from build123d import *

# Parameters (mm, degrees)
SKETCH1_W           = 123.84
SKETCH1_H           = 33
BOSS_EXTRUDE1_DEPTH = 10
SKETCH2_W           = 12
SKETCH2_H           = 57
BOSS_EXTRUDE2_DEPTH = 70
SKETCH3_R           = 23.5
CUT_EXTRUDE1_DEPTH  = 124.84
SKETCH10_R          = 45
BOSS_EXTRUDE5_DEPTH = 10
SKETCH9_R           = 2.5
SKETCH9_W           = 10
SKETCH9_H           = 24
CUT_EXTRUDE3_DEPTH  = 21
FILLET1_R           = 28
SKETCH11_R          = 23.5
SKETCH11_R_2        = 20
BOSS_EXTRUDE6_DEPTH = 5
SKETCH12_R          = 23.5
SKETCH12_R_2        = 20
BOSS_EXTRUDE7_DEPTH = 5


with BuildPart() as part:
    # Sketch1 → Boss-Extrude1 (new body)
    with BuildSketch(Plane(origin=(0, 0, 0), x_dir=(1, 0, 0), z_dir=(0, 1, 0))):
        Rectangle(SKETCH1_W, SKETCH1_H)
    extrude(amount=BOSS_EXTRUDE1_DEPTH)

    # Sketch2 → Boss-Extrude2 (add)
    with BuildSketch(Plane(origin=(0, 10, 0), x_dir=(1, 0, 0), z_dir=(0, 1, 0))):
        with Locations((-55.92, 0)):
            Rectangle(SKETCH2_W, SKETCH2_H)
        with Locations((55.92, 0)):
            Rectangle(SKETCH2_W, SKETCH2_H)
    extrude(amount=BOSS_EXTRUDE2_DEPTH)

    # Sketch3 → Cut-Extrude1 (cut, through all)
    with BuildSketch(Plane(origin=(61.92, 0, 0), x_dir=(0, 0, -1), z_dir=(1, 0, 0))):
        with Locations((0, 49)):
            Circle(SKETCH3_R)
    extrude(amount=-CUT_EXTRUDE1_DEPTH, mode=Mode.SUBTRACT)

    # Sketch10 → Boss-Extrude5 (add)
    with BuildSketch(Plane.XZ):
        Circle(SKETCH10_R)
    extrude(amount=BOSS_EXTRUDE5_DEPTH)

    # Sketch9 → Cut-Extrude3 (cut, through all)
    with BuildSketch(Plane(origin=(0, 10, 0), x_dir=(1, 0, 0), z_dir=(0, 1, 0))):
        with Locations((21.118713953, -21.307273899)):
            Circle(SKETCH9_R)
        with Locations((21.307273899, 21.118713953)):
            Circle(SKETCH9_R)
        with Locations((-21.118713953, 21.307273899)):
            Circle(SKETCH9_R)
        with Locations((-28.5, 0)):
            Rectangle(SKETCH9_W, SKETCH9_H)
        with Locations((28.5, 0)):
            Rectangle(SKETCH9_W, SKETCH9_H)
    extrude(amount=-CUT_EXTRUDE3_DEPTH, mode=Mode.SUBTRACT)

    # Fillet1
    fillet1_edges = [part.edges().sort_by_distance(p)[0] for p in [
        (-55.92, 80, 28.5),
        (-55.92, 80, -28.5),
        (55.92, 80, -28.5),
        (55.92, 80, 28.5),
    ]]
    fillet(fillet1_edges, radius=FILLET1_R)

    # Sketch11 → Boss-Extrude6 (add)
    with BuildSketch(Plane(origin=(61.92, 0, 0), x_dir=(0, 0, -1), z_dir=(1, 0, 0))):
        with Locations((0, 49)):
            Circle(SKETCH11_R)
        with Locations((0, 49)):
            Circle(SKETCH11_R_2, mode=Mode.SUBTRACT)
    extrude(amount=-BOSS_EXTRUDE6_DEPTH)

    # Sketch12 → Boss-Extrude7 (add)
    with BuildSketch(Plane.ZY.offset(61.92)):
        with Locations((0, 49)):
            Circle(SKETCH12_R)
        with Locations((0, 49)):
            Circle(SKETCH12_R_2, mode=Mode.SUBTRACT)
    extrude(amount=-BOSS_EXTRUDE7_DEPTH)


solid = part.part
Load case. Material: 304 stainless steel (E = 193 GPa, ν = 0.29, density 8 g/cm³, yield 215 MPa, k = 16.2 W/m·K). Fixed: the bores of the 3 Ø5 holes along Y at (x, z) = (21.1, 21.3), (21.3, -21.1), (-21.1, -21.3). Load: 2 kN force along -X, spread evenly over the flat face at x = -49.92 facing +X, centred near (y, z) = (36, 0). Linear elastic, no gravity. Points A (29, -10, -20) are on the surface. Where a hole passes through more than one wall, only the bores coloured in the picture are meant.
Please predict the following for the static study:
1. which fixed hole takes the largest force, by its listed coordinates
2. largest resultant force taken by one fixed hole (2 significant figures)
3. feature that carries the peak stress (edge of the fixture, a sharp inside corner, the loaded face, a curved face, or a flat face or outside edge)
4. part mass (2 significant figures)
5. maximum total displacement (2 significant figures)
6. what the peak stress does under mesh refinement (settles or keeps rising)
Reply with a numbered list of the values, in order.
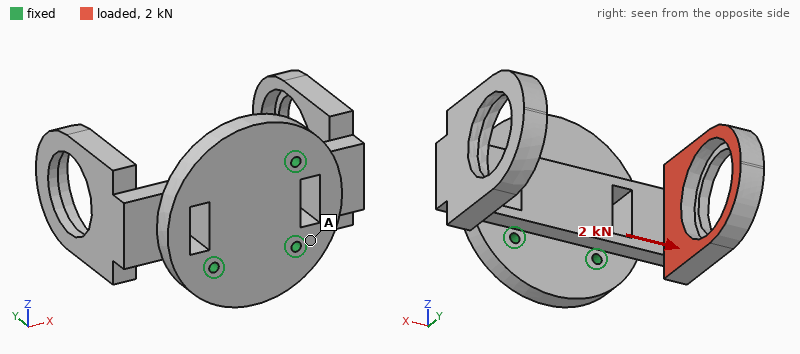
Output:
1. (21.3, -21.1)
2. 1.9 kN
3. edge of the fixture
4. 1.2 kg
5. 0.33 mm
6. keeps rising
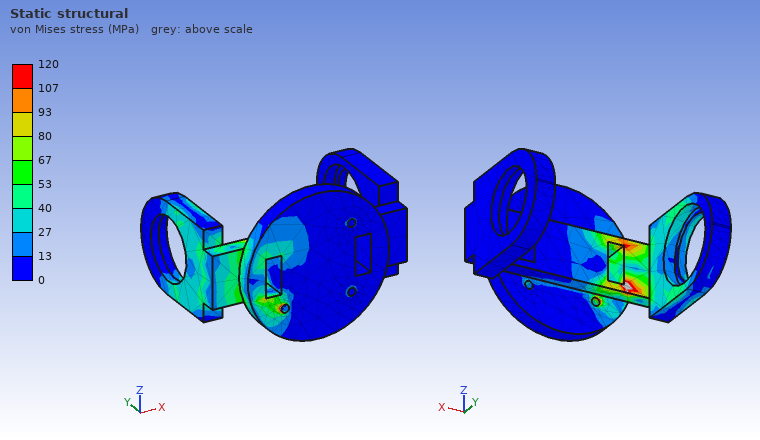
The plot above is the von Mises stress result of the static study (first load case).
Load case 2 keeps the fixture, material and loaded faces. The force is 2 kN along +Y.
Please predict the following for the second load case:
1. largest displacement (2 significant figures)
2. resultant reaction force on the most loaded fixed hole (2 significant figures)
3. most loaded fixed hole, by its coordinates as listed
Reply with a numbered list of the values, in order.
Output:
1. 72 µm
2. 2.8 kN
3. (-21.1, -21.3)
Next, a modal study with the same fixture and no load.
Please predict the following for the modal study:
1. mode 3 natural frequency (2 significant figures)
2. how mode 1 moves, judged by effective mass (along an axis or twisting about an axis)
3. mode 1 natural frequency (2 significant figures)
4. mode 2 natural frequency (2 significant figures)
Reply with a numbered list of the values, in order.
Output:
1. 1400 Hz
2. along X
3. 1000 Hz
4. 1100 Hz
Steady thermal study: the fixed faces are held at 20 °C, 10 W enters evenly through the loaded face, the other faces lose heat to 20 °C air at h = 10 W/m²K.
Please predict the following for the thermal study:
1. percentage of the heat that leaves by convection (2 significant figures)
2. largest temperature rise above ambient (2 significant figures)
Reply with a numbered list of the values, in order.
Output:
1. 54 %
2. 68 K
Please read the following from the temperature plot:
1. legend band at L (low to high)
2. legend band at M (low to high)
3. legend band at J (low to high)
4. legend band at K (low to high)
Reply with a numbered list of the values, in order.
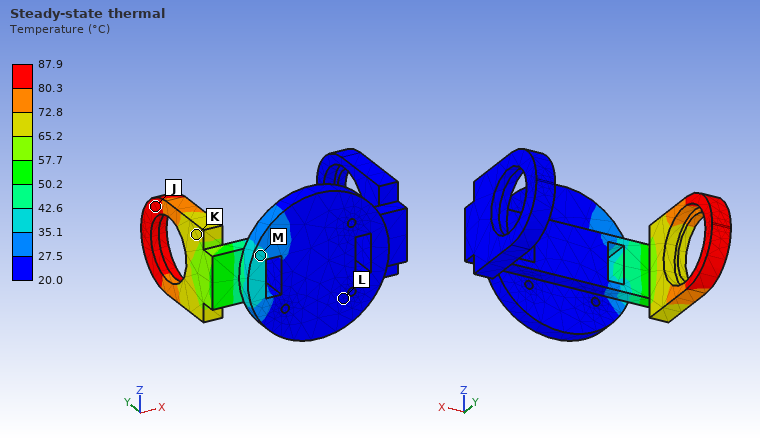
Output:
1. 20.0 to 27.5 °C
2. 35.1 to 42.6 °C
3. 80.3 to 87.9 °C
4. 65.2 to 72.8 °C
